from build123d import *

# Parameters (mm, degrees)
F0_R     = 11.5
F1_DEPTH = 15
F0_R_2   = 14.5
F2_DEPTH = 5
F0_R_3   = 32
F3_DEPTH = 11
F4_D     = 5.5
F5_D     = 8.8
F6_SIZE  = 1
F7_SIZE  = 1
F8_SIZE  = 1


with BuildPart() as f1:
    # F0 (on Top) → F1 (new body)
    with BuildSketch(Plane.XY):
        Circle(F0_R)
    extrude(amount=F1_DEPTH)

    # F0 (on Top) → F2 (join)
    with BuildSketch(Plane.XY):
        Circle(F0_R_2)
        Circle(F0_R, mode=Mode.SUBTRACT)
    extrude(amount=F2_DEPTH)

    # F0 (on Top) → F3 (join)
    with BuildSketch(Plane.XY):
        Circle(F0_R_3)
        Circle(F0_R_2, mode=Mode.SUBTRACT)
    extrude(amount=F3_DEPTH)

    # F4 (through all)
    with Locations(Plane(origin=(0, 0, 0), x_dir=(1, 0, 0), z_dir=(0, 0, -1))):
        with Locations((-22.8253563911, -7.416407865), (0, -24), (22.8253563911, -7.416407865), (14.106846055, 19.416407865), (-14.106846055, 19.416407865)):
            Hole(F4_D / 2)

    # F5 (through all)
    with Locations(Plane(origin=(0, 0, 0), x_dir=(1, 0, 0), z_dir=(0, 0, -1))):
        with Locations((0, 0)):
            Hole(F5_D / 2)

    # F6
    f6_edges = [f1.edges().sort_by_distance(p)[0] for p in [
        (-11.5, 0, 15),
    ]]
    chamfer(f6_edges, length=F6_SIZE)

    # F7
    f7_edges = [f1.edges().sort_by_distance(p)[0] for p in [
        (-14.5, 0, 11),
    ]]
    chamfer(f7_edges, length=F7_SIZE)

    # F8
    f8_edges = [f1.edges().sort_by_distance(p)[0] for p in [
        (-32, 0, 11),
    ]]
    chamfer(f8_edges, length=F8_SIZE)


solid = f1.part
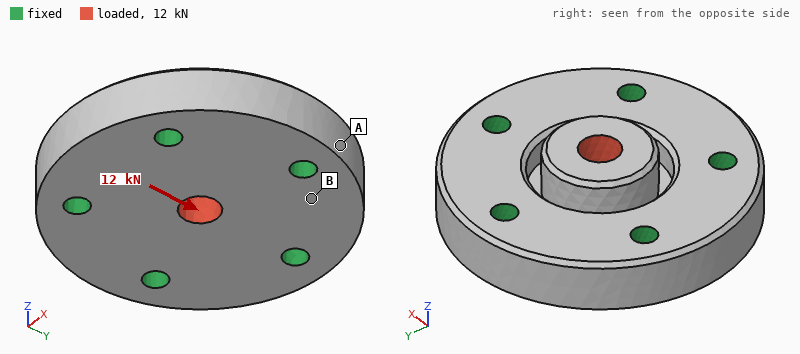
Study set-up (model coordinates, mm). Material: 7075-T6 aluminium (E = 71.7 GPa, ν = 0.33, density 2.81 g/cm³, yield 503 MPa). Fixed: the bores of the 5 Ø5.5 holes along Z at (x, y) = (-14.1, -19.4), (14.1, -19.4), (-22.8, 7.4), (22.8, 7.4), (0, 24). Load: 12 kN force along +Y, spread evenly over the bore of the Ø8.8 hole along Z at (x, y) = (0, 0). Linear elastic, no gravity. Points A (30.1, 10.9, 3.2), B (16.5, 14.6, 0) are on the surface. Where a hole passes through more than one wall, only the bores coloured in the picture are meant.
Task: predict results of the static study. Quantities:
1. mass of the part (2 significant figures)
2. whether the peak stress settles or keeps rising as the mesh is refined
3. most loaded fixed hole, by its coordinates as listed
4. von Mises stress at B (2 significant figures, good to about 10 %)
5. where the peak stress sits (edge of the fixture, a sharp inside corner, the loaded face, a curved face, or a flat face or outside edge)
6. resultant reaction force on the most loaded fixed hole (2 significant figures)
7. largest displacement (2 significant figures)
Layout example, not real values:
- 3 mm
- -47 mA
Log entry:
- 93 g
- keeps rising
- (0, 24)
- 20 MPa
- edge of the fixture
- 3.5 kN
- 31 µm
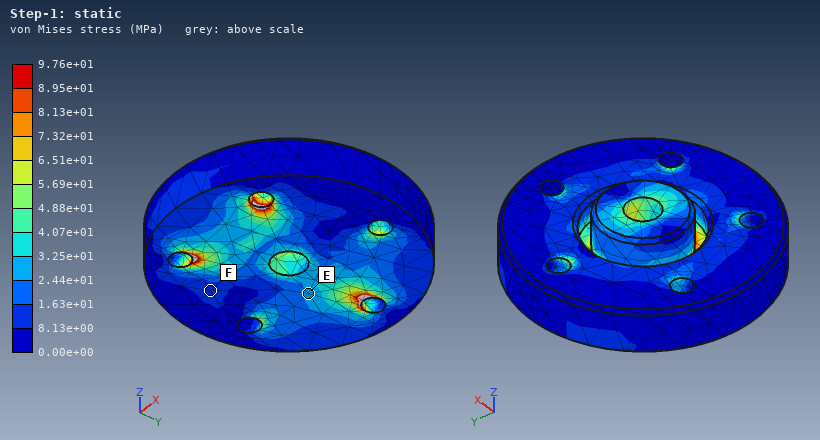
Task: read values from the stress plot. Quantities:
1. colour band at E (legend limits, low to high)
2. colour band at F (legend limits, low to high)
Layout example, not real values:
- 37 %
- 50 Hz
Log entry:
- 2.44e+01 to 3.25e+01 MPa
- 8.13e+00 to 1.63e+01 MPa
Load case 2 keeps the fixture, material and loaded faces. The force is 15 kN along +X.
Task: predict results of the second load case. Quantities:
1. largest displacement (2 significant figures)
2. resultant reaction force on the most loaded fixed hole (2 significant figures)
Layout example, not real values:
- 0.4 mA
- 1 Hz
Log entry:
- 38 µm
- 4.2 kN
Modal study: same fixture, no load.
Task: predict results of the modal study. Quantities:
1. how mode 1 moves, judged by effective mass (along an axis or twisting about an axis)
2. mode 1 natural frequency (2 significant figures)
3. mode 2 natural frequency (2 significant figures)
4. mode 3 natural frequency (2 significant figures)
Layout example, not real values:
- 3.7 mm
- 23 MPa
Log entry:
- along Z
- 25 kHz
- 28 kHz
- 28 kHz
